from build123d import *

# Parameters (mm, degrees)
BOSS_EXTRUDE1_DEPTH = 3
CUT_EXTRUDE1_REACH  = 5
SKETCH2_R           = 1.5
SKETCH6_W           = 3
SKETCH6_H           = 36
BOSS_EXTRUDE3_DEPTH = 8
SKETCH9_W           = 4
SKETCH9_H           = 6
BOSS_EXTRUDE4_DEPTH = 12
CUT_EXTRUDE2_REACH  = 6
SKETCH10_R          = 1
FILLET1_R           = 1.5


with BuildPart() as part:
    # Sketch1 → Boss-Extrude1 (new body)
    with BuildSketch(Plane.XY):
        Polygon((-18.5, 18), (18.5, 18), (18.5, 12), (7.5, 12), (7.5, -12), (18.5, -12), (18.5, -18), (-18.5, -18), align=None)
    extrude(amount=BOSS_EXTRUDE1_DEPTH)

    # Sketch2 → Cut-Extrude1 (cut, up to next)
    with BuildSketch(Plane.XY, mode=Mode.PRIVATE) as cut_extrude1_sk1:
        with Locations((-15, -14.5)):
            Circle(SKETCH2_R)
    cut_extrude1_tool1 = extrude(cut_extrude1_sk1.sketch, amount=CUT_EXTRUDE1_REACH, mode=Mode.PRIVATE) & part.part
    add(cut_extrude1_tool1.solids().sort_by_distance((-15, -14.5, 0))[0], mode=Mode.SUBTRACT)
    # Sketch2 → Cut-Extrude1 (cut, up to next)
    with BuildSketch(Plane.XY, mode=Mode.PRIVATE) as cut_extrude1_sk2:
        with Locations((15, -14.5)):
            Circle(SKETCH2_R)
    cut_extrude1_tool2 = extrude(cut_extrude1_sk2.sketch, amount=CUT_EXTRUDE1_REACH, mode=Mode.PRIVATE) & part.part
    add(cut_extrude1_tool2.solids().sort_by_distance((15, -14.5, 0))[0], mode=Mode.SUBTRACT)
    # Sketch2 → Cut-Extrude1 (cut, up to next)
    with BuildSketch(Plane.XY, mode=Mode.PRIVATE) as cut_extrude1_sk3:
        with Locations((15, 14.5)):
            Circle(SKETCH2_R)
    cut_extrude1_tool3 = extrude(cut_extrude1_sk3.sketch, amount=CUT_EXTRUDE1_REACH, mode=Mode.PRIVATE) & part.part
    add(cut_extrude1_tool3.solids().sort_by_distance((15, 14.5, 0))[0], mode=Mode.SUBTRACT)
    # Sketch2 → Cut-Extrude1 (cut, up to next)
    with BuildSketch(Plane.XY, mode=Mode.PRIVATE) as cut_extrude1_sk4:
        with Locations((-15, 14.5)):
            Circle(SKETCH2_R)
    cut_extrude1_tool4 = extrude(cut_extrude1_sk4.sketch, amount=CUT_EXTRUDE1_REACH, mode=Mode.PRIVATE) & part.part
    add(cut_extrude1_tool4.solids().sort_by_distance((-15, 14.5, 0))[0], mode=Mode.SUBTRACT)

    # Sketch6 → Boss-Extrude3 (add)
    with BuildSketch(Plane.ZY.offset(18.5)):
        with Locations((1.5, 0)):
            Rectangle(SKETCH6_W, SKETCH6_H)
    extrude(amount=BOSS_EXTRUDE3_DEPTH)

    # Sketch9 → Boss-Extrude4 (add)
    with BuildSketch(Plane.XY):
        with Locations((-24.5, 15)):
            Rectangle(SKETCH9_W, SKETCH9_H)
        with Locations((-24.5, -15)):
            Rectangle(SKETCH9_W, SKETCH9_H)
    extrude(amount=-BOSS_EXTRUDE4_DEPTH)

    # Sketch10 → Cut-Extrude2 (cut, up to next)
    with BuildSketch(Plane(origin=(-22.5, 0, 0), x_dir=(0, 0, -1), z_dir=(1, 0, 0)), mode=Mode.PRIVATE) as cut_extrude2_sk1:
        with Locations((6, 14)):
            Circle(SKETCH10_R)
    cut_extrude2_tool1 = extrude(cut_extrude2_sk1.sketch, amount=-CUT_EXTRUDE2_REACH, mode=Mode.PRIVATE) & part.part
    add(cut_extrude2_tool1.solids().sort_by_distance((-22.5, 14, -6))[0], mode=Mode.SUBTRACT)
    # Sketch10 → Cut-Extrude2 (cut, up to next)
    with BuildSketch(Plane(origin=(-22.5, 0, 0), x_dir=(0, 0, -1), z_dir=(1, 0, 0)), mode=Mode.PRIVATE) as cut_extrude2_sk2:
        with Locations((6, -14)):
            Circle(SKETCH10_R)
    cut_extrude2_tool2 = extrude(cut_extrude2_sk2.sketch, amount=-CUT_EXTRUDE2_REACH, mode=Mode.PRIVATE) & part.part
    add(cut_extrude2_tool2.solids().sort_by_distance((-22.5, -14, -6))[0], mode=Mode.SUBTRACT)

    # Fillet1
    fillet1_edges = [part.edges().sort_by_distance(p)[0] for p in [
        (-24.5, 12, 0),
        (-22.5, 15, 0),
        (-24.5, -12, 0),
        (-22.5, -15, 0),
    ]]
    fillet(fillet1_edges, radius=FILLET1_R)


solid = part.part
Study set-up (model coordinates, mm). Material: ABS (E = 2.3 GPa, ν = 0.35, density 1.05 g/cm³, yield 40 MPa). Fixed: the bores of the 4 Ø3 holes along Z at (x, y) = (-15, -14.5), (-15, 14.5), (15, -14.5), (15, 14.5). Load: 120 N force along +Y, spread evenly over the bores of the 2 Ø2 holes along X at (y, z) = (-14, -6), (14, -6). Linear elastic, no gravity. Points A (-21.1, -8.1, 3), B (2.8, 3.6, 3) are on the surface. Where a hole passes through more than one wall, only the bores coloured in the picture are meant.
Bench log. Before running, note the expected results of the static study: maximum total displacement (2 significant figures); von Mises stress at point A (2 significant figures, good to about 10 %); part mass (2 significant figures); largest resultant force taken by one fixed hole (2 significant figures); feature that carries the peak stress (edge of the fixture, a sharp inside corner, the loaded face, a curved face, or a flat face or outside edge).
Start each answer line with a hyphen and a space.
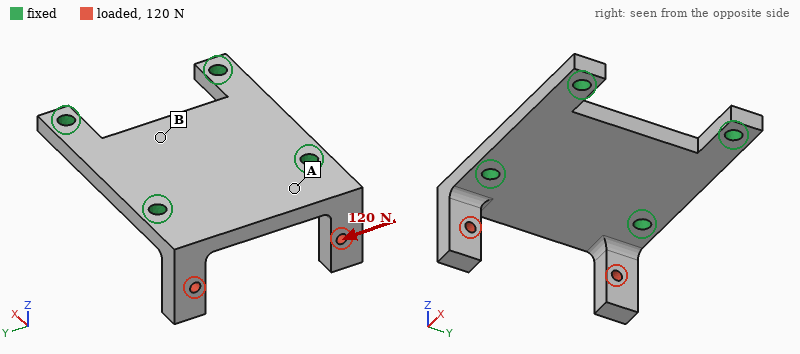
- 0.54 mm
- 7.1 MPa
- 4.8 g
- 71 N
- a curved face
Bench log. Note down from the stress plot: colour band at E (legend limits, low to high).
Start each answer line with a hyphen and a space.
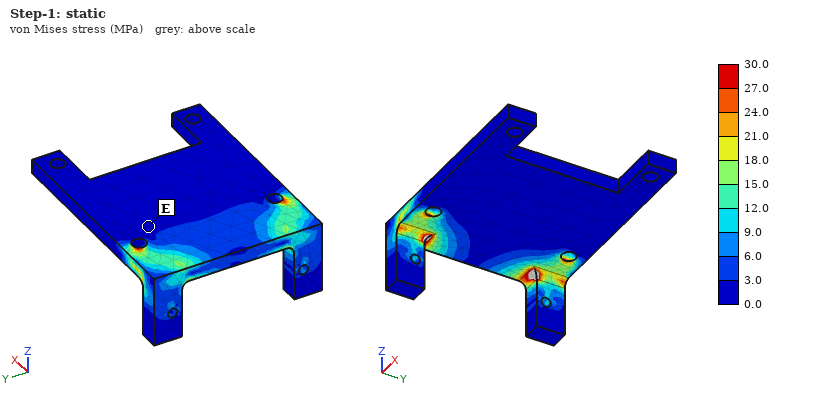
- 0.0 to 3.0 MPa
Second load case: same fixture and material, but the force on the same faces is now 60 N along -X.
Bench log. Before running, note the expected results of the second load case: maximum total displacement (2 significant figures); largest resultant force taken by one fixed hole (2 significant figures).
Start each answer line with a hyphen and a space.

- 0.52 mm
- 29 N
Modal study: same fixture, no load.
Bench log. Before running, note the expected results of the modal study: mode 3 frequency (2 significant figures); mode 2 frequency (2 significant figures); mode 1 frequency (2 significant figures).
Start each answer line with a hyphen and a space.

- 3000 Hz
- 2500 Hz
- 2300 Hz
